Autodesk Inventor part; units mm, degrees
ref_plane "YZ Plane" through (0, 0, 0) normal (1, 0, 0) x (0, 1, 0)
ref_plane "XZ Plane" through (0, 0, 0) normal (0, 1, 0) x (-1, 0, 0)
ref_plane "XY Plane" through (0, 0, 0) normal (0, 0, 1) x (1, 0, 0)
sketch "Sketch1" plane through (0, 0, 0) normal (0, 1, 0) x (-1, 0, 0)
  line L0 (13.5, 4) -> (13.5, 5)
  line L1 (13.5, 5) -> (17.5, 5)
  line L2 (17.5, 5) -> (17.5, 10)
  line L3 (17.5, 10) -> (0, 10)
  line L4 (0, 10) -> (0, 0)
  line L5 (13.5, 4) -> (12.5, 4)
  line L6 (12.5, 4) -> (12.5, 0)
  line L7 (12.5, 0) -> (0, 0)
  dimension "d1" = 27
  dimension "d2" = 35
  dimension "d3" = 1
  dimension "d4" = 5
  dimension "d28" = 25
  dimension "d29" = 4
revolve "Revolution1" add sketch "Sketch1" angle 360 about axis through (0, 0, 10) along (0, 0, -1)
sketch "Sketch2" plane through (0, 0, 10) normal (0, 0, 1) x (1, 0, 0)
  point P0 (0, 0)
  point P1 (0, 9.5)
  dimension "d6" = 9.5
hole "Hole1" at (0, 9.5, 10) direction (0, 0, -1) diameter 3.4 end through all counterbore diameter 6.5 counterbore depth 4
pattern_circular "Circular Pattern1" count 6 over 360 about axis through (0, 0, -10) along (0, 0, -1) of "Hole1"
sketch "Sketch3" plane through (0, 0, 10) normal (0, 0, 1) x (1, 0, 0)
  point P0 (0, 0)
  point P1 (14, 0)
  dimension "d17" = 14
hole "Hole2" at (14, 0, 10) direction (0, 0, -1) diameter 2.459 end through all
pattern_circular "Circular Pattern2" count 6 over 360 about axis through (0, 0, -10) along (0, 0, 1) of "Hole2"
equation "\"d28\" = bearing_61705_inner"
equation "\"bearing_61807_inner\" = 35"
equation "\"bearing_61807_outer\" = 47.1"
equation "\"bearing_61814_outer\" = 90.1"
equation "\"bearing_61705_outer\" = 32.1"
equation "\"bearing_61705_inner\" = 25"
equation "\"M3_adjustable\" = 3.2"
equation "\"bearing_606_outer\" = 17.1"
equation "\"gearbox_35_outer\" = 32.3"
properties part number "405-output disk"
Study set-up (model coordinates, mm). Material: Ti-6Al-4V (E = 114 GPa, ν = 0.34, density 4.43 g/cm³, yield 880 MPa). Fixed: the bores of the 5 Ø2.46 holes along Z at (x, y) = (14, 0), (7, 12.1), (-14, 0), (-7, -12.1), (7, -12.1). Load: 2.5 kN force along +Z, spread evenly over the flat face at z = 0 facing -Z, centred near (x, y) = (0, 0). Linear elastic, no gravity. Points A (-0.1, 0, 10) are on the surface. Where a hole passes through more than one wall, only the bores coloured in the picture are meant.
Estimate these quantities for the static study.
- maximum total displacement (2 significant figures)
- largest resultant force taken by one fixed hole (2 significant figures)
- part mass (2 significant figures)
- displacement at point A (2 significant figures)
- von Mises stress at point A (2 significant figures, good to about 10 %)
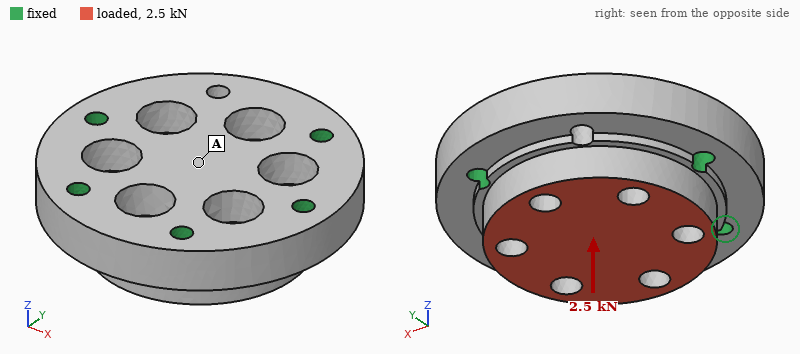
3.8 µm
730 N
27 g
2.3 µm
8.6 MPa
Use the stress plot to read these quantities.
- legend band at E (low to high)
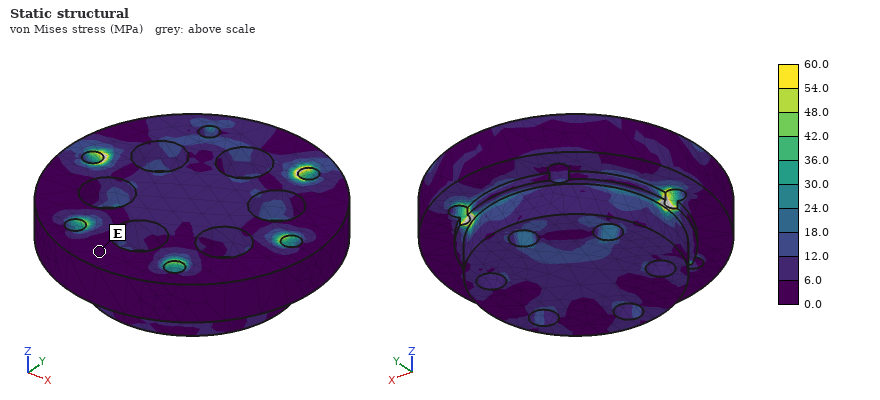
0.0 to 6.0 MPa
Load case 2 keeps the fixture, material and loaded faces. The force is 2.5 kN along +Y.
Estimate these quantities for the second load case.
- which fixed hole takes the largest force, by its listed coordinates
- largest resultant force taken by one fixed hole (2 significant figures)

(7, 12.1)
850 N
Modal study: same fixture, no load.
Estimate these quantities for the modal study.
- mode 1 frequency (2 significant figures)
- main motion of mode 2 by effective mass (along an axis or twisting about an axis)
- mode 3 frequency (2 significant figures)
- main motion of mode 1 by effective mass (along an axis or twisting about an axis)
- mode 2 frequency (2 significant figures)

29 kHz
along Z
53 kHz
along Z
47 kHz
